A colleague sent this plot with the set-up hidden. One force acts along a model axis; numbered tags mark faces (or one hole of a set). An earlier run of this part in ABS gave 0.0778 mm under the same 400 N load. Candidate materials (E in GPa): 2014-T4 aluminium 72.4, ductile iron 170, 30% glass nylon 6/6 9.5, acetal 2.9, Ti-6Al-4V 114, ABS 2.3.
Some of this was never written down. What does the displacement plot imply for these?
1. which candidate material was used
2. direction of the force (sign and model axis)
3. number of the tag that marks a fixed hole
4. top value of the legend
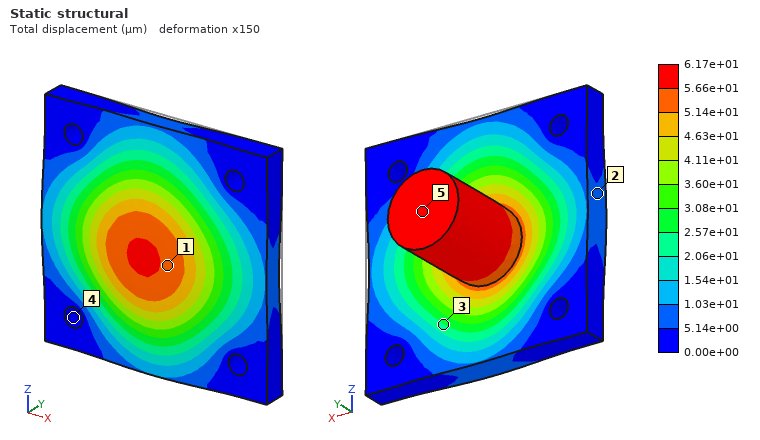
acetal
-Y
4
6.17e+01 µm
